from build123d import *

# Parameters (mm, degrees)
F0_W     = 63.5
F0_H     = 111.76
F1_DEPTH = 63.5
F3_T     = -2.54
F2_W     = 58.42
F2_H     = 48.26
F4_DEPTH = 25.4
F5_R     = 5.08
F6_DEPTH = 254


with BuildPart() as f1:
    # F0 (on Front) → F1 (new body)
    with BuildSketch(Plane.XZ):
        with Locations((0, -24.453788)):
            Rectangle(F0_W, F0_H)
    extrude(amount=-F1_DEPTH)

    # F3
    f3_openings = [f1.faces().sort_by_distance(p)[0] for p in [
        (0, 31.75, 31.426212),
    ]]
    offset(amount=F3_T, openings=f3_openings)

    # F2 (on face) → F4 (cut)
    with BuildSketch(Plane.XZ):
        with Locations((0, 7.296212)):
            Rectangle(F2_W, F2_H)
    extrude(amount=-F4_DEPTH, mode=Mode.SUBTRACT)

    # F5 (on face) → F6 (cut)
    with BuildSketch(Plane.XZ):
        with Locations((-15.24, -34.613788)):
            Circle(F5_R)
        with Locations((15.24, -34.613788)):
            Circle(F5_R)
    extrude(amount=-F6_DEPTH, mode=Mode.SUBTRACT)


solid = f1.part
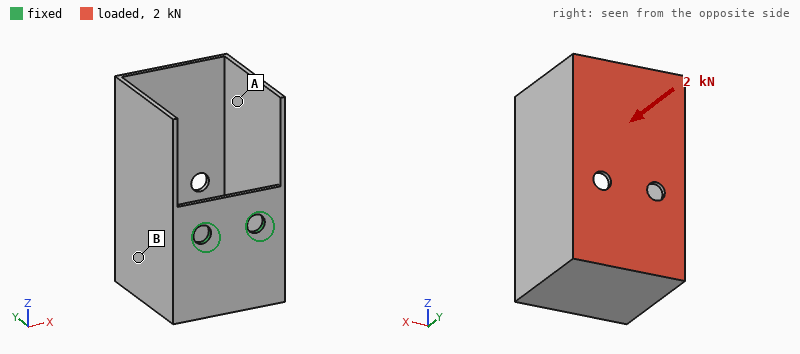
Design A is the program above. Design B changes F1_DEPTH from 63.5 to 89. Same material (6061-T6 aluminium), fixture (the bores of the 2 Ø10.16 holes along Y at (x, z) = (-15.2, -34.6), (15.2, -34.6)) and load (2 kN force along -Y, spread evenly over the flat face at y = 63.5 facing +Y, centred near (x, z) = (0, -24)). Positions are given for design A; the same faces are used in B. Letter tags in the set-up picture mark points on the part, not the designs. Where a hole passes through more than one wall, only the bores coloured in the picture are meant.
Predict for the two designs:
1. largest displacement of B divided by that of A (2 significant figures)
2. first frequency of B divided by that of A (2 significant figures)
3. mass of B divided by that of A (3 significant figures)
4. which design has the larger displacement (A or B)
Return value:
1.1
0.71
1.26
B
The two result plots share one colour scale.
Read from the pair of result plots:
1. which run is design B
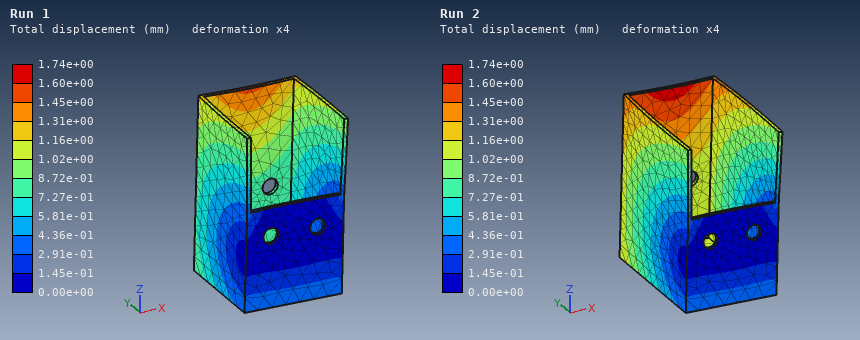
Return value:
Run 2
